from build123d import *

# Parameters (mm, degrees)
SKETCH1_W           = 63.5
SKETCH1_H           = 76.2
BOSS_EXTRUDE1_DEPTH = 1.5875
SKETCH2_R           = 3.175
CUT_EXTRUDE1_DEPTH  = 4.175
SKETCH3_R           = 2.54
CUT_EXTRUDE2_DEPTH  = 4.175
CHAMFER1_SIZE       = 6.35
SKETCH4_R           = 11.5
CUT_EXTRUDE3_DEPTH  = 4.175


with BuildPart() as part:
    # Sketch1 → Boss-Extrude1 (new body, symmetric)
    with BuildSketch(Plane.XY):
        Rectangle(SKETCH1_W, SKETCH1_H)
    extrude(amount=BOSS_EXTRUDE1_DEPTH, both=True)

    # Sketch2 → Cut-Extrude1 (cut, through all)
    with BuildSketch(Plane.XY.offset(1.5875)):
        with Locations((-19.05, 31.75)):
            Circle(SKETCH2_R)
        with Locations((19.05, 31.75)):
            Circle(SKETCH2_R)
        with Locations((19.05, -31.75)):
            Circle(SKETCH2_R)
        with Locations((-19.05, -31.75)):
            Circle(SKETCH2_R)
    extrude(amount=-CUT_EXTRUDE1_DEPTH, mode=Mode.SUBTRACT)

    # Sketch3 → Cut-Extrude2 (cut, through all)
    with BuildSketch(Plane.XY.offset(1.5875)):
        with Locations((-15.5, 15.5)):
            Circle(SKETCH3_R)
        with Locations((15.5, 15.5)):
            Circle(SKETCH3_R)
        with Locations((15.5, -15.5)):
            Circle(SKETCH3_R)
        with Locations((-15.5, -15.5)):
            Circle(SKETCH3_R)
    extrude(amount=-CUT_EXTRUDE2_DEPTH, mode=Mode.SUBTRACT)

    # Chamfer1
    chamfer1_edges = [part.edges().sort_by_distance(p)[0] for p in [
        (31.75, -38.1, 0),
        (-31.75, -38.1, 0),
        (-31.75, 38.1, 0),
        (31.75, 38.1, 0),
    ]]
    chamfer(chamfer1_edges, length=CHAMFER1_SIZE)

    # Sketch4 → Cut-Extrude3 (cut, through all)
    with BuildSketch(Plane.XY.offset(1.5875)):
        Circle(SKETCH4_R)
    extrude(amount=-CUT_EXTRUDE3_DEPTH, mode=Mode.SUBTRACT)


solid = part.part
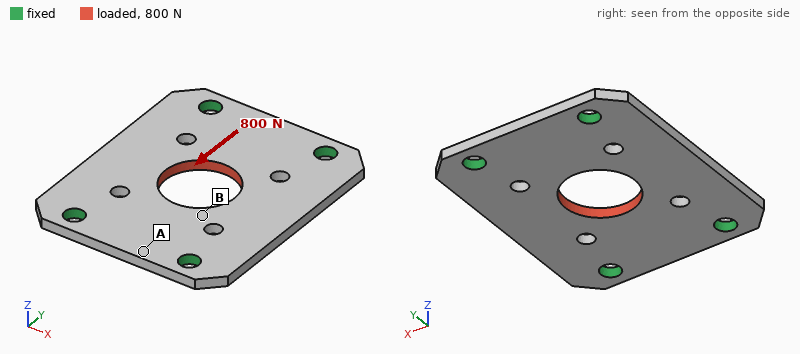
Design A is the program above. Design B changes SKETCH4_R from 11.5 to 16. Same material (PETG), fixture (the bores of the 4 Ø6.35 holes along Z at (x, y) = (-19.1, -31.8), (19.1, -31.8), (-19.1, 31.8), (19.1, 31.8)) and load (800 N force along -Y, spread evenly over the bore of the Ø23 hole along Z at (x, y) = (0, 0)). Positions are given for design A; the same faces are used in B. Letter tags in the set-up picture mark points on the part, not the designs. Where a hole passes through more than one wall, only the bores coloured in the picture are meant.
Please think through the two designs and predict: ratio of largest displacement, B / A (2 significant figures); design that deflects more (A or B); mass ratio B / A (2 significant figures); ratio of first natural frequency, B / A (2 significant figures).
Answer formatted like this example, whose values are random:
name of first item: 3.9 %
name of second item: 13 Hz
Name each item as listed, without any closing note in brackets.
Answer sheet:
ratio of largest displacement, B / A: 0.85
design that deflects more: A
mass ratio B / A: 0.91
ratio of first natural frequency, B / A: 1.1
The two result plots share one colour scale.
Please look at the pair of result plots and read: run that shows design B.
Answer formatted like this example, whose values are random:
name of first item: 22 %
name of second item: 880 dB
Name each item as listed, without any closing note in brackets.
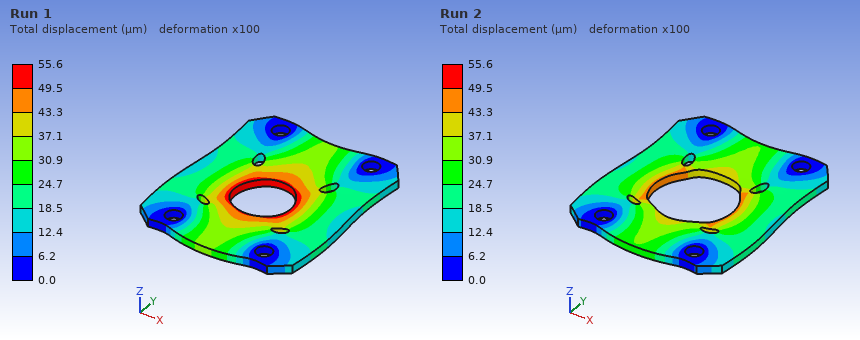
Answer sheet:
run that shows design B: Run 2
